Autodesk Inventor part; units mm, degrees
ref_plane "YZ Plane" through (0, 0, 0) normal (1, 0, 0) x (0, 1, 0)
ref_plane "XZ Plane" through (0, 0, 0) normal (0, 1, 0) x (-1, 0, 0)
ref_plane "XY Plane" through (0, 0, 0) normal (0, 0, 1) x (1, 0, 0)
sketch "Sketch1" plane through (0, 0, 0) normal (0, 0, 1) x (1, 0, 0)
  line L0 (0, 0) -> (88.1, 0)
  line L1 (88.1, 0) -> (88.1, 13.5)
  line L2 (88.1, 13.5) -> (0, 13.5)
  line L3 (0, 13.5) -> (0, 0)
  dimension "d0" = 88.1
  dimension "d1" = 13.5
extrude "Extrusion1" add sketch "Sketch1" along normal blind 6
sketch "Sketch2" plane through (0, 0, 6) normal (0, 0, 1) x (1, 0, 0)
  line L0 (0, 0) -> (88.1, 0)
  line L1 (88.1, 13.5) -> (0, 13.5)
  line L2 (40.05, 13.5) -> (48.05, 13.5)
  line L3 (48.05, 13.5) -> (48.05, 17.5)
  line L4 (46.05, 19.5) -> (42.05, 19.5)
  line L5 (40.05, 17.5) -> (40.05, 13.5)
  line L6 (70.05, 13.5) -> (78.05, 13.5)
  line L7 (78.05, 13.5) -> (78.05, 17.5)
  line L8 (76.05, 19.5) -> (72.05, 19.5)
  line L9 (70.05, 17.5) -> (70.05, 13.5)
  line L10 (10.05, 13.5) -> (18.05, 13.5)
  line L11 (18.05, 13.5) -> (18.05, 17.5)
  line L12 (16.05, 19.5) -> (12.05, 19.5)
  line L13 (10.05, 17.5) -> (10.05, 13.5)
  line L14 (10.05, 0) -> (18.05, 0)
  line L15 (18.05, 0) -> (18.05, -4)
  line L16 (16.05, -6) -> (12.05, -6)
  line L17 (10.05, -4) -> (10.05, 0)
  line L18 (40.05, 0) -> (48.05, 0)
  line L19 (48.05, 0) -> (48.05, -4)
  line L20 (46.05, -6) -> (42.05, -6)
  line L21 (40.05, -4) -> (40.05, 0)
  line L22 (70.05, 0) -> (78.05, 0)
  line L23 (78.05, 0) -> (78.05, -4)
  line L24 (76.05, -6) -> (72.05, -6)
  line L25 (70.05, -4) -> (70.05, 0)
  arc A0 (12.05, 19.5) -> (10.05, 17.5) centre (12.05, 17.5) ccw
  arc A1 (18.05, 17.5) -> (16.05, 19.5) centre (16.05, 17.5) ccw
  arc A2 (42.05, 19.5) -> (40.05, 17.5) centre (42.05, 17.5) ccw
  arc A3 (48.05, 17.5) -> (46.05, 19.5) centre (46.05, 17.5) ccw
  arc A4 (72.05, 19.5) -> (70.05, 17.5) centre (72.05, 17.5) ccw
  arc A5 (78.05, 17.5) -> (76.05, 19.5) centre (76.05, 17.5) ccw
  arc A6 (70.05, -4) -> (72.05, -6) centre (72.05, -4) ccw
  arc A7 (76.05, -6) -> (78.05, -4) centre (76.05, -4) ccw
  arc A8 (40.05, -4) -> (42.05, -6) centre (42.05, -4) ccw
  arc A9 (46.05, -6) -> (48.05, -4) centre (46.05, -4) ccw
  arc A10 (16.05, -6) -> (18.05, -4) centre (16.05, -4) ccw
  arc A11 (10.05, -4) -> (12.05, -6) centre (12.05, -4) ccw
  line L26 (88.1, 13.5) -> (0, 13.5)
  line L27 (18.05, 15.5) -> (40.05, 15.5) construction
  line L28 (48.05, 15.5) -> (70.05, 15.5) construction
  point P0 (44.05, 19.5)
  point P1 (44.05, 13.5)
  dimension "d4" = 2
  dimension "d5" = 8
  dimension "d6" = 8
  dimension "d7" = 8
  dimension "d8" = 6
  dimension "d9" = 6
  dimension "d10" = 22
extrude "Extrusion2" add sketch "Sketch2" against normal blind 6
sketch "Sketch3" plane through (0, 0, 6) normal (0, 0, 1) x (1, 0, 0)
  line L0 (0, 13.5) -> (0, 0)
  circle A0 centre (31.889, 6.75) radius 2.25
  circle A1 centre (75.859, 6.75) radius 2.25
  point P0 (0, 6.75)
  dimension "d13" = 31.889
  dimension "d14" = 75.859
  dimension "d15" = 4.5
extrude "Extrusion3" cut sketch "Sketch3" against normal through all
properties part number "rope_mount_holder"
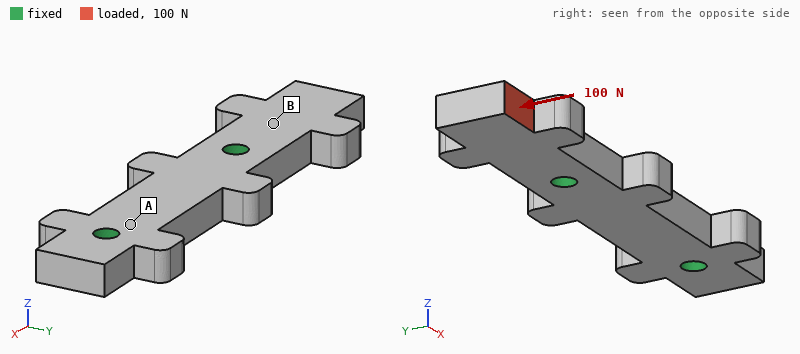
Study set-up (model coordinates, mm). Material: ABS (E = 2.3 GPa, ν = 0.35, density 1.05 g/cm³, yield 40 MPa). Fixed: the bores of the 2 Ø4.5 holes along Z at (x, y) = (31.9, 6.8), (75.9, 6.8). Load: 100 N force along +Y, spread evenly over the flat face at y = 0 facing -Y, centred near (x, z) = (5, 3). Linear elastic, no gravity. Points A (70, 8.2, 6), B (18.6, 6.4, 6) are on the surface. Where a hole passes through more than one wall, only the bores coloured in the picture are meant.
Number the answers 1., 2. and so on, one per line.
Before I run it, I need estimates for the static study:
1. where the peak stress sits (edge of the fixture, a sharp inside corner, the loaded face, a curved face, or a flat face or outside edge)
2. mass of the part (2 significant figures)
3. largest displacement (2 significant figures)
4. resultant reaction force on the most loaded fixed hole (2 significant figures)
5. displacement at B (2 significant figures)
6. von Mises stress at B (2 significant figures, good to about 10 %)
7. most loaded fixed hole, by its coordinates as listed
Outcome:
1. edge of the fixture
2. 9.0 g
3. 0.47 mm
4. 130 N
5. 0.14 mm
6. 3.9 MPa
7. (31.9, 6.8)
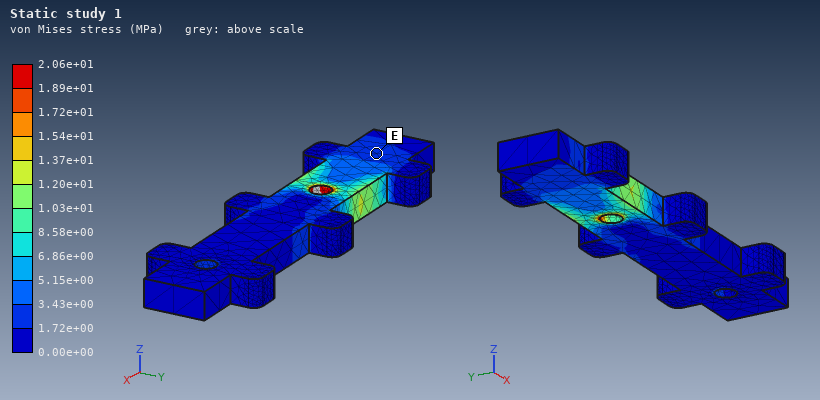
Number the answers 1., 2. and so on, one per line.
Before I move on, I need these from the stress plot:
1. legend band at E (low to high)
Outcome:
1. 1.72e+00 to 3.43e+00 MPa
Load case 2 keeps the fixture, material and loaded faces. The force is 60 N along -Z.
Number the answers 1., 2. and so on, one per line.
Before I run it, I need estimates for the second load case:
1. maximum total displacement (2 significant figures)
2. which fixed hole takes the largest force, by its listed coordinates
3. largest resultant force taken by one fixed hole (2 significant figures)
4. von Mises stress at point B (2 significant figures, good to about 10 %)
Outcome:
1. 0.94 mm
2. (31.9, 6.8)
3. 62 N
4. 10 MPa
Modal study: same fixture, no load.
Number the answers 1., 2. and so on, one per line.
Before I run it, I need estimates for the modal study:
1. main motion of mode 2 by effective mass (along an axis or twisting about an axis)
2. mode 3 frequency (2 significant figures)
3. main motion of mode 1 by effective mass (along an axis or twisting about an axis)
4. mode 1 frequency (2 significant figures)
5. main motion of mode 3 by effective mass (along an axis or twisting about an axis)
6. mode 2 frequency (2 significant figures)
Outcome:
1. along Y
2. 3300 Hz
3. along Z
4. 1400 Hz
5. twisting about X
6. 2100 Hz
